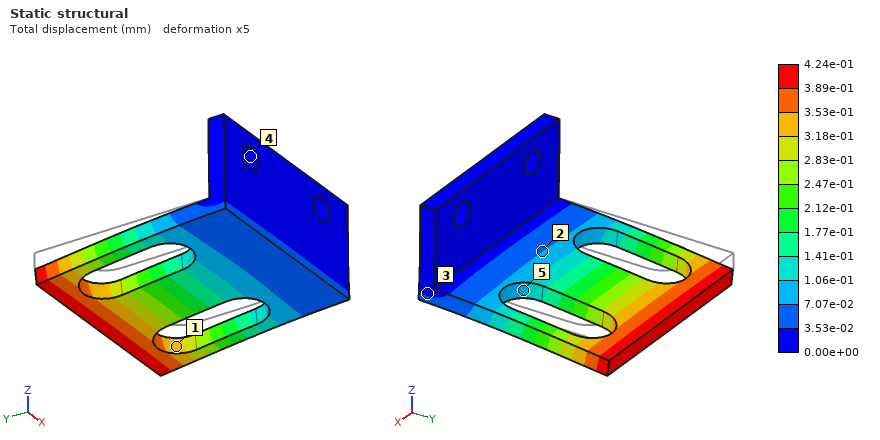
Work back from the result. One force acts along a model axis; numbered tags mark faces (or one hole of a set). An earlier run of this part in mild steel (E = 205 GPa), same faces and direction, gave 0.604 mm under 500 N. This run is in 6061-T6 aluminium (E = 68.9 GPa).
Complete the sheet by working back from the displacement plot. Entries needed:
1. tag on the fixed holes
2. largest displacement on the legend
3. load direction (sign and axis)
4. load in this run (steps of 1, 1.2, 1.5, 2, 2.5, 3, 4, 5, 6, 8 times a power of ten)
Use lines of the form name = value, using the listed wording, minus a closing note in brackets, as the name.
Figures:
tag on the fixed holes = 4
largest displacement on the legend = 4.24e-01 mm
load direction = -Z
load in this run = 120 N
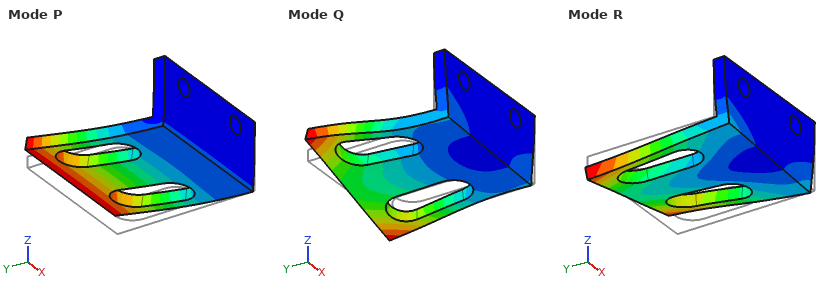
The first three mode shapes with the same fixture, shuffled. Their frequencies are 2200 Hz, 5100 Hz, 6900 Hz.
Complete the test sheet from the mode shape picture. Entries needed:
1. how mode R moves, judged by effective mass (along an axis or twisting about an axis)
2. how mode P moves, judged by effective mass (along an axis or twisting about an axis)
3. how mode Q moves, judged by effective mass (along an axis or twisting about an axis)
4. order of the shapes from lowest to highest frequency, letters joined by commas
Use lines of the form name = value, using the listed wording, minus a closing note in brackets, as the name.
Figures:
how mode R moves, judged by effective mass = along X
how mode P moves, judged by effective mass = along Z
how mode Q moves, judged by effective mass = along X
order of the shapes from lowest to highest frequency, letters joined by commas = P, R, Q
